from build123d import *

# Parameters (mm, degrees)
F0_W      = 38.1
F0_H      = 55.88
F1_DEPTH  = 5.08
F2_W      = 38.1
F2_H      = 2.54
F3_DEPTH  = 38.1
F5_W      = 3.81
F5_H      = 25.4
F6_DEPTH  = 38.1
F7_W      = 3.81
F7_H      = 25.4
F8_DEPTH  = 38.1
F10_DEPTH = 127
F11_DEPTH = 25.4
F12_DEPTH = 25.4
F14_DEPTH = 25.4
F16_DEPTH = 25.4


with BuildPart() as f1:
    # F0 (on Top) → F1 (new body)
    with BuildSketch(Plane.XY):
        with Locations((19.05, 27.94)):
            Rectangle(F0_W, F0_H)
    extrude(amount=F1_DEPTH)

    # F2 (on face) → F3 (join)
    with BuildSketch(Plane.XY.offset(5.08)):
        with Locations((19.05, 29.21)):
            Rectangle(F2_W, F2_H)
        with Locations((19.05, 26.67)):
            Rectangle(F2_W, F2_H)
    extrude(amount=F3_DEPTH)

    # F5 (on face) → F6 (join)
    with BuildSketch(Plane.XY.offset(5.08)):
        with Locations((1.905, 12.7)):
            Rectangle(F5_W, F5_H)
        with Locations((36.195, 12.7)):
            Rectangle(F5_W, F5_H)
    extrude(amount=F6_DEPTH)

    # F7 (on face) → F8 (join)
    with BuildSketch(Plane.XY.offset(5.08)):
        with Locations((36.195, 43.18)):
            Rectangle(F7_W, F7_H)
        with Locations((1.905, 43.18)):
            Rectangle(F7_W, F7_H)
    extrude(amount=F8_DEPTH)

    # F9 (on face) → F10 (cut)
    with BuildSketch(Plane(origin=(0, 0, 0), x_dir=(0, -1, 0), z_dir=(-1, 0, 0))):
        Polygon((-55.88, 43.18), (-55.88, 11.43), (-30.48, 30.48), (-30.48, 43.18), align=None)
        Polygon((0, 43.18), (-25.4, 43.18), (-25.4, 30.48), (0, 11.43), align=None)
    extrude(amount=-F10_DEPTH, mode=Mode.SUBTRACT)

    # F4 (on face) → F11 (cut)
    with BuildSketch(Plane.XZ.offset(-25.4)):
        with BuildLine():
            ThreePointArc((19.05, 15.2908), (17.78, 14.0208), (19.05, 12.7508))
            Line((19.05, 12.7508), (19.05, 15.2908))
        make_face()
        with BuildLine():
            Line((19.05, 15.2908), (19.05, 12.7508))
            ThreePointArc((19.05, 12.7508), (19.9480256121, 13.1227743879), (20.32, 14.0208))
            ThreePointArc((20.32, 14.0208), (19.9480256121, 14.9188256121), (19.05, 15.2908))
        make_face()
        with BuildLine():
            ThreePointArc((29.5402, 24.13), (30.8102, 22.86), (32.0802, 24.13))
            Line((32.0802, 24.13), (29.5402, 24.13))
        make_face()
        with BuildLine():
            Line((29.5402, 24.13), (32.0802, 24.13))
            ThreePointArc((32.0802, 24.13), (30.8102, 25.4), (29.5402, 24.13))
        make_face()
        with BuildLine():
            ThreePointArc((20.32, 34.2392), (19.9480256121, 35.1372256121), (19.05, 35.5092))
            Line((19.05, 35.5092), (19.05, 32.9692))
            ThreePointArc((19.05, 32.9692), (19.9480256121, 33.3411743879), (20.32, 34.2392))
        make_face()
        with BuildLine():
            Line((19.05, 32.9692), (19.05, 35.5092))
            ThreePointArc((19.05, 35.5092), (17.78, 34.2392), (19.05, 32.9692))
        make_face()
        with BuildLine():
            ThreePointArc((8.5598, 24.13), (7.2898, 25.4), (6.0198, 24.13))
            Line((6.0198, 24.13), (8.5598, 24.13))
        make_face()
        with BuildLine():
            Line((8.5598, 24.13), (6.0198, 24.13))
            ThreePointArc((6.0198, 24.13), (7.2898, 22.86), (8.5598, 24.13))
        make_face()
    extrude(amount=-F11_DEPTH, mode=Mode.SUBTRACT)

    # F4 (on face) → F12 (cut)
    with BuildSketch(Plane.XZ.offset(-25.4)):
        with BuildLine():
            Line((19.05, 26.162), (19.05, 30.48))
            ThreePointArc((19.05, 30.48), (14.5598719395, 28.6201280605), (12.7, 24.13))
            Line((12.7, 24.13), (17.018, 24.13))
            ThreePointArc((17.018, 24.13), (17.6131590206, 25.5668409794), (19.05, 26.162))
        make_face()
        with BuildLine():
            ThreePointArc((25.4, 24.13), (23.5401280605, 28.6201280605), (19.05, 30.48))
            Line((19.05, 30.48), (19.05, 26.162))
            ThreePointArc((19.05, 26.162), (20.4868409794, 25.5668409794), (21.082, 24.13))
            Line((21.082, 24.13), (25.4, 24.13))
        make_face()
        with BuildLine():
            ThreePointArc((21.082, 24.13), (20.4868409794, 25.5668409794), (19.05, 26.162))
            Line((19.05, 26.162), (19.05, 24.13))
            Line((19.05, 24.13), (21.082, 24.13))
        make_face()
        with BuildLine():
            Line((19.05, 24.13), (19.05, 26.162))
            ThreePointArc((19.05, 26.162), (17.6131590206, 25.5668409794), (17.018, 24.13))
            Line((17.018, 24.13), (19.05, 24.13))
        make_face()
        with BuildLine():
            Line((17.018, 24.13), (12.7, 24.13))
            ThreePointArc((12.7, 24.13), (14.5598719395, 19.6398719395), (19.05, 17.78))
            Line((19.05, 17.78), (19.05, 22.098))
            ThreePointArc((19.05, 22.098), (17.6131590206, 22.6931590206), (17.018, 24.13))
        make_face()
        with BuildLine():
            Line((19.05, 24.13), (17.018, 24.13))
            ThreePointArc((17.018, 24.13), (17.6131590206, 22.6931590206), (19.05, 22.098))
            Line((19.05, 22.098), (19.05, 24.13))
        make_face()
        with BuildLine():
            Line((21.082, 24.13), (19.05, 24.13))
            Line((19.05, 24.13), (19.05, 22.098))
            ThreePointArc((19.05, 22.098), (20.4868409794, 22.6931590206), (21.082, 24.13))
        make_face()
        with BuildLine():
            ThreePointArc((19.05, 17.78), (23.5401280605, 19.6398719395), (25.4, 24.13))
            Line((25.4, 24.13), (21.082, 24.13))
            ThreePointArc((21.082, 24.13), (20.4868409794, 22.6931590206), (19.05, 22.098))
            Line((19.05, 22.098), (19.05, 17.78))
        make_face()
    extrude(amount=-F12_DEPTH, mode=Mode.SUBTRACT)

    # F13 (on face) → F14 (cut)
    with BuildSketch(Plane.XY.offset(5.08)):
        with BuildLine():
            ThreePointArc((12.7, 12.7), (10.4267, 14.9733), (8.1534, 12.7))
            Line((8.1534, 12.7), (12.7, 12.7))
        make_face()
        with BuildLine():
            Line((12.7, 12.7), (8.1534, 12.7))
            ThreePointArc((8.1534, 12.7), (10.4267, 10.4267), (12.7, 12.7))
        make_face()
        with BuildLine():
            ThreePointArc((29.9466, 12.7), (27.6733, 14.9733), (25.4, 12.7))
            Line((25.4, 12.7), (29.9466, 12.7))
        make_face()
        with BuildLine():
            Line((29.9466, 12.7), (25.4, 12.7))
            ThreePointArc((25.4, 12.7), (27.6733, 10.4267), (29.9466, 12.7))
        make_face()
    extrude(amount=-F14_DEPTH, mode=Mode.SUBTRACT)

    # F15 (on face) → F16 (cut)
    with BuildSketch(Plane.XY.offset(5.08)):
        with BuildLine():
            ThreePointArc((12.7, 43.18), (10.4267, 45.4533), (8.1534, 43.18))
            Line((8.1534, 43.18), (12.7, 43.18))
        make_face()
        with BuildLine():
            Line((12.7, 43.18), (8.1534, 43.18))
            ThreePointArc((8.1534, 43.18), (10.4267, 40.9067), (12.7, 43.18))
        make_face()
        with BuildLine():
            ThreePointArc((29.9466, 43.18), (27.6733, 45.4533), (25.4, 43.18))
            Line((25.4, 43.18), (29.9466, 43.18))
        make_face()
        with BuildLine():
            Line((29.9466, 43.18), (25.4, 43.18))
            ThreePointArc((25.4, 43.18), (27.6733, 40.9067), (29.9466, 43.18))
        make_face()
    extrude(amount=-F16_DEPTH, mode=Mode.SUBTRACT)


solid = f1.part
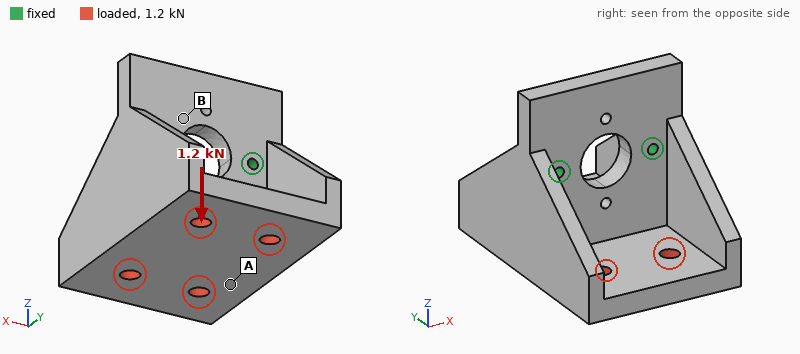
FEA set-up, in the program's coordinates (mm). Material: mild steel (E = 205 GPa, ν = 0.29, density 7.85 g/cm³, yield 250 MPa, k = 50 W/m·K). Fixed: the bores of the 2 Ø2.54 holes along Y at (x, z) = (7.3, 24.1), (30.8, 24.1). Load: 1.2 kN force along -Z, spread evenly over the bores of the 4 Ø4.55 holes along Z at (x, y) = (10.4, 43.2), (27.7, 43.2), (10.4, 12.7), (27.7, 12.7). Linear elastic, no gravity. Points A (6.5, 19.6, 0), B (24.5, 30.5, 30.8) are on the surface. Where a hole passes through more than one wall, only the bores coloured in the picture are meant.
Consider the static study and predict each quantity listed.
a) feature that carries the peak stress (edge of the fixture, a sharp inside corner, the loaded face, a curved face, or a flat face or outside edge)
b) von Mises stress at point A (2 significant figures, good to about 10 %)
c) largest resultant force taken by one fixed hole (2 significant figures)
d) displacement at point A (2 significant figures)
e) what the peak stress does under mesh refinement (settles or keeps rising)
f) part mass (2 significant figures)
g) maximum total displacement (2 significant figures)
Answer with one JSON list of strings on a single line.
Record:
["edge of the fixture", "9.9 MPa", "610 N", "1.2 µm", "keeps rising", "180 g", "3.9 µm"]
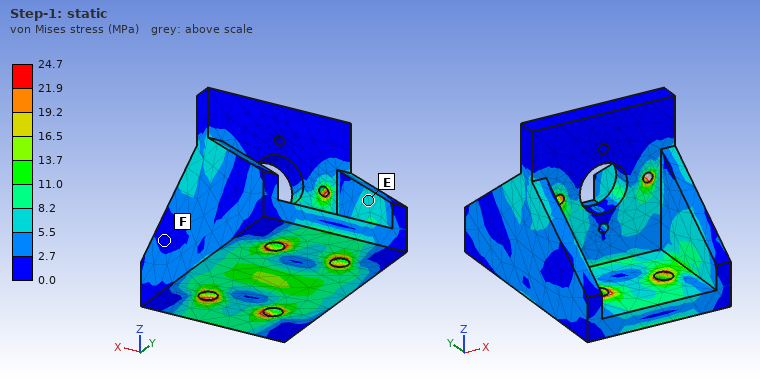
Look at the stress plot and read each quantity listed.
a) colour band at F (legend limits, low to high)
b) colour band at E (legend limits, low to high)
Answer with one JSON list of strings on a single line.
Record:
["0.0 to 2.7 MPa", "5.5 to 8.2 MPa"]
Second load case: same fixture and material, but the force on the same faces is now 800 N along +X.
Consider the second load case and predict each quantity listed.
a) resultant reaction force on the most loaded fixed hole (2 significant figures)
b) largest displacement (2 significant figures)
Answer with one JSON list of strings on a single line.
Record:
["780 N", "3.4 µm"]
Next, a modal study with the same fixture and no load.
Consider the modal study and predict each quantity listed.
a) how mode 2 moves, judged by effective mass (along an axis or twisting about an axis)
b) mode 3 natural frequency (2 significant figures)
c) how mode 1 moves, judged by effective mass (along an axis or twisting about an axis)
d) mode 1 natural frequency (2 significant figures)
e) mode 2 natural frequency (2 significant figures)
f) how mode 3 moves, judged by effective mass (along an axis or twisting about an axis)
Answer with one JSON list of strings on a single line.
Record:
["twisting about Z", "7600 Hz", "along Y", "2300 Hz", "3700 Hz", "along X"]
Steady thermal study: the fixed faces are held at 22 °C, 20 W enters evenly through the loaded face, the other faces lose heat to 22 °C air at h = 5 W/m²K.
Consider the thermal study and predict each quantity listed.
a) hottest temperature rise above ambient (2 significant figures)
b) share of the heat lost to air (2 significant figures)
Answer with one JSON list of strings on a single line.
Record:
["39 K", "6.8 %"]
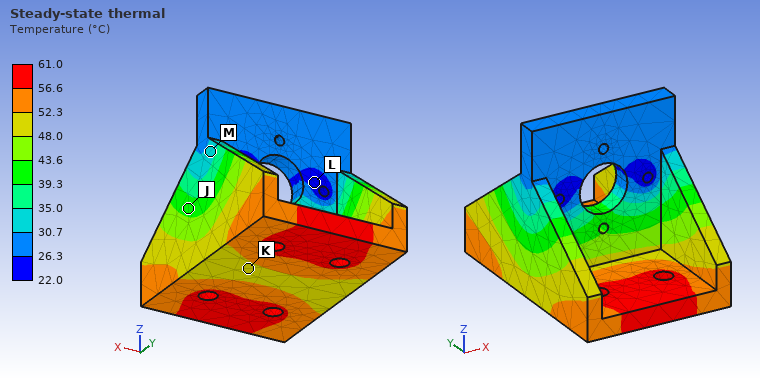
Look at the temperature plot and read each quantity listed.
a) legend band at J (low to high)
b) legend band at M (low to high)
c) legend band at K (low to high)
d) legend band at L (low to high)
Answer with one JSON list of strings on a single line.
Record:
["39.3 to 43.6 °C", "30.7 to 35.0 °C", "48.0 to 52.3 °C", "22.0 to 26.3 °C"]
